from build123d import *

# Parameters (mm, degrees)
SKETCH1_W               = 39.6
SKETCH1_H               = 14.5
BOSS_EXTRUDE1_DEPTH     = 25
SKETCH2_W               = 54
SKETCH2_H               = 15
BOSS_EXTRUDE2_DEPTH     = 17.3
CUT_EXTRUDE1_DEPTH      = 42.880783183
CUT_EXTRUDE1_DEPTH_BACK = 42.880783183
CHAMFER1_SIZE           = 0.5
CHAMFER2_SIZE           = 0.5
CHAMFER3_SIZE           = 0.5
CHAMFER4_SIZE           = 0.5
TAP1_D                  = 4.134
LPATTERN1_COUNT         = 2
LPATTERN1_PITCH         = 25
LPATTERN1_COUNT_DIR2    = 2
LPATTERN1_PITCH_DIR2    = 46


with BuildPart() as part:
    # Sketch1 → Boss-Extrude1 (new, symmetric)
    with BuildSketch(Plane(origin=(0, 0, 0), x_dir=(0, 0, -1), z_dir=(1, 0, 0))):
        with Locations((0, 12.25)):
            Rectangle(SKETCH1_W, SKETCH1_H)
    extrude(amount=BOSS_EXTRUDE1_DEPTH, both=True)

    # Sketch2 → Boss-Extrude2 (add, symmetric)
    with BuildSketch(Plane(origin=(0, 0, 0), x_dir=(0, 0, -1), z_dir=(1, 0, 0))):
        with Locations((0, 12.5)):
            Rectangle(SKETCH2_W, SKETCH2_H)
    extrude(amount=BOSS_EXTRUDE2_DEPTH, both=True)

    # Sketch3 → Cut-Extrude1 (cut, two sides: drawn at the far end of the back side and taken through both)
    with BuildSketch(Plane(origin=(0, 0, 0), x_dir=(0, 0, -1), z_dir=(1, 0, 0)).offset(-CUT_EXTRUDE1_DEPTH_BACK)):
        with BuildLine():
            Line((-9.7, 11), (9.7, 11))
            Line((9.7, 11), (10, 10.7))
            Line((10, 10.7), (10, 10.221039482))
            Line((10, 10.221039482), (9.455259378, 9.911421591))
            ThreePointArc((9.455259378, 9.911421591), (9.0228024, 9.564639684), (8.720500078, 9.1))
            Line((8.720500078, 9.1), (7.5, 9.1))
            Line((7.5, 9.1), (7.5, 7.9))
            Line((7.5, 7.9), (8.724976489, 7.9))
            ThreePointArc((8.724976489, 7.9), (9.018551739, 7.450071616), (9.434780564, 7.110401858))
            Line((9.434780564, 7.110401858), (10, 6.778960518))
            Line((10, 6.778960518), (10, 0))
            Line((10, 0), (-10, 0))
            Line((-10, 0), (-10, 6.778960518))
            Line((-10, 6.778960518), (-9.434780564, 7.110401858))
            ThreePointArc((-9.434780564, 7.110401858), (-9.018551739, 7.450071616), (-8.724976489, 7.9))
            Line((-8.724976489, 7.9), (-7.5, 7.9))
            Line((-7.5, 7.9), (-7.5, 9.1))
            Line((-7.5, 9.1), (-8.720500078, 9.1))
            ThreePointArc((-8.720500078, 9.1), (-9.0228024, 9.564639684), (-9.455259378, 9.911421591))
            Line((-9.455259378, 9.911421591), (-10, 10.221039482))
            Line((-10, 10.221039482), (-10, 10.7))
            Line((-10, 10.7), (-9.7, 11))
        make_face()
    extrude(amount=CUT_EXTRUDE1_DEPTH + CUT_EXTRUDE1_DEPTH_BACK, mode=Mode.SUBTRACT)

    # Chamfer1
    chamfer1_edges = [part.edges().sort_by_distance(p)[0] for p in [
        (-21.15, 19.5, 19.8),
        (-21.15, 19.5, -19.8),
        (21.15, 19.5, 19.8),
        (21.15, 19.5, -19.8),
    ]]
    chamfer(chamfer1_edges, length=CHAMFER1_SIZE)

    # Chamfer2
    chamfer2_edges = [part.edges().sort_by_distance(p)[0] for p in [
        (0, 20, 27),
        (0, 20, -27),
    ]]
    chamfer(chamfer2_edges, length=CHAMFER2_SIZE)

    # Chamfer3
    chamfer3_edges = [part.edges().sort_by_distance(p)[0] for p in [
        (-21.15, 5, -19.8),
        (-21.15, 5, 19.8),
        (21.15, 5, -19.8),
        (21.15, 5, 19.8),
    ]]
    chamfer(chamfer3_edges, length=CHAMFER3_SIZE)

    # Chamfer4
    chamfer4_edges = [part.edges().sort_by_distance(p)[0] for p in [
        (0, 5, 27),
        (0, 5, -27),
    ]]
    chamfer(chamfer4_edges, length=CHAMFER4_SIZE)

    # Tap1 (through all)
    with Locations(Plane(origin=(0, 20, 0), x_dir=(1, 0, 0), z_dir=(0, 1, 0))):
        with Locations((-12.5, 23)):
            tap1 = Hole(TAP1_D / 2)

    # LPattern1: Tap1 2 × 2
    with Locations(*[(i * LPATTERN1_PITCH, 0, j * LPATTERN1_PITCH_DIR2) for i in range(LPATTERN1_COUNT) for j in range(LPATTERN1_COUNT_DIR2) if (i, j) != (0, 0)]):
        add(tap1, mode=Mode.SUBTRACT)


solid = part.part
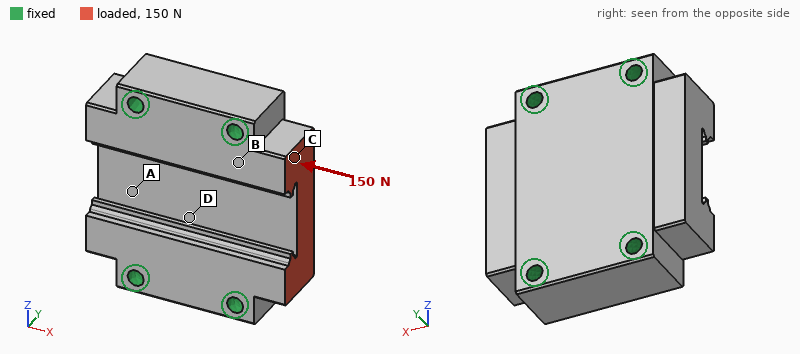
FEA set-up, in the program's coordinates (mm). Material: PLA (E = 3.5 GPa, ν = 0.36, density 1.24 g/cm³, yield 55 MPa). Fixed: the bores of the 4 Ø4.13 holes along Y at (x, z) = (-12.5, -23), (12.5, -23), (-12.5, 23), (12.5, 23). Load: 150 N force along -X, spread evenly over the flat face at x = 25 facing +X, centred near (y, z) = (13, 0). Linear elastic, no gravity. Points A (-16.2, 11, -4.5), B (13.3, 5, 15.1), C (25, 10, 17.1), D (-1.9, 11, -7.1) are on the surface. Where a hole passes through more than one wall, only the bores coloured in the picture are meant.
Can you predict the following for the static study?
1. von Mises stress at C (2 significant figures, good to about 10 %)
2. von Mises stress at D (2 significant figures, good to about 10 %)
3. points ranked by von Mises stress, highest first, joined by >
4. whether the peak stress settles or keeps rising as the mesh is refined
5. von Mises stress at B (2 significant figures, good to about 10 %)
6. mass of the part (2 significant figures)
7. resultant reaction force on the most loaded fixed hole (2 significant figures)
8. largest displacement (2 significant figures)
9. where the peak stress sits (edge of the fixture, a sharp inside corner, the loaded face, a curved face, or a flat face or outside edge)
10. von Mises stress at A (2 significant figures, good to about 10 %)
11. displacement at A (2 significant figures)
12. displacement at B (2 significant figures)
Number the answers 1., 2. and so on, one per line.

1. 0.35 MPa
2. 0.17 MPa
3. C > B > D > A
4. keeps rising
5. 0.26 MPa
6. 38 g
7. 47 N
8. 3.3 µm
9. edge of the fixture
10. 0.072 MPa
11. 0.98 µm
12. 1.3 µm
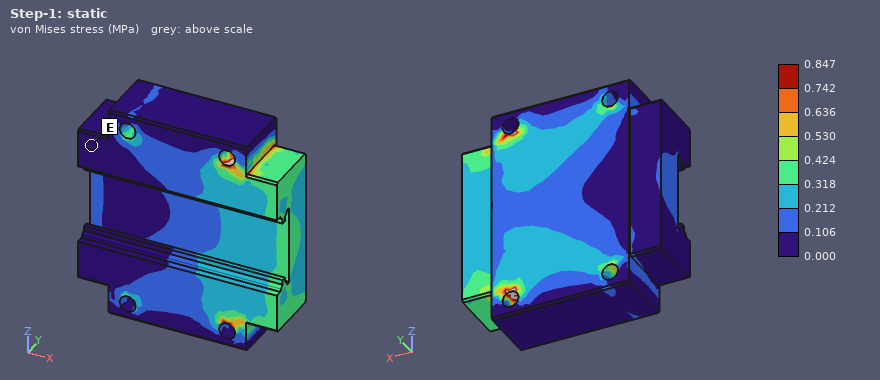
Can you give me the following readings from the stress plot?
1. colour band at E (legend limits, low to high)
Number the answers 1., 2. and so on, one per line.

1. 0.000 to 0.106 MPa
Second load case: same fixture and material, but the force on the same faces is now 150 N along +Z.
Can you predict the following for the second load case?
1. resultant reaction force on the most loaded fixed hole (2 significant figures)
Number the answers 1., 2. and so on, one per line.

1. 80 N
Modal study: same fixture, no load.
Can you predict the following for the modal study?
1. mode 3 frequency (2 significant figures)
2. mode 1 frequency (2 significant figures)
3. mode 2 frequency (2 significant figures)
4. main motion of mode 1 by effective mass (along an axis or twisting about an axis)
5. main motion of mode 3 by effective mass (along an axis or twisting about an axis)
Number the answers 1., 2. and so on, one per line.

1. 9900 Hz
2. 6700 Hz
3. 7200 Hz
4. along Y
5. along X
